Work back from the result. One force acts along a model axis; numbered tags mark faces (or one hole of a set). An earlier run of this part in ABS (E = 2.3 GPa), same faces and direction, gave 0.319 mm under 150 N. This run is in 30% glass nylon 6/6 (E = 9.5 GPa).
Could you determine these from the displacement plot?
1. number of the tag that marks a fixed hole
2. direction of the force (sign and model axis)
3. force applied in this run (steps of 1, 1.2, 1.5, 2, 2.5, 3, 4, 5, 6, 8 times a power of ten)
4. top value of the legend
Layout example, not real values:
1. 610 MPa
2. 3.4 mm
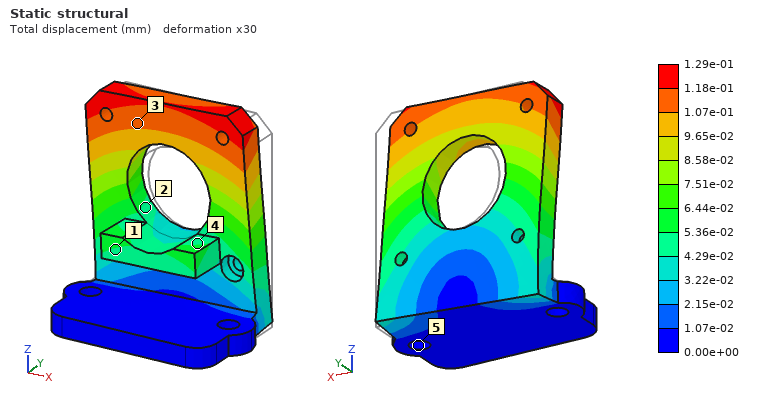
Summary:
1. 5
2. -X
3. 250 N
4. 1.29e-01 mm
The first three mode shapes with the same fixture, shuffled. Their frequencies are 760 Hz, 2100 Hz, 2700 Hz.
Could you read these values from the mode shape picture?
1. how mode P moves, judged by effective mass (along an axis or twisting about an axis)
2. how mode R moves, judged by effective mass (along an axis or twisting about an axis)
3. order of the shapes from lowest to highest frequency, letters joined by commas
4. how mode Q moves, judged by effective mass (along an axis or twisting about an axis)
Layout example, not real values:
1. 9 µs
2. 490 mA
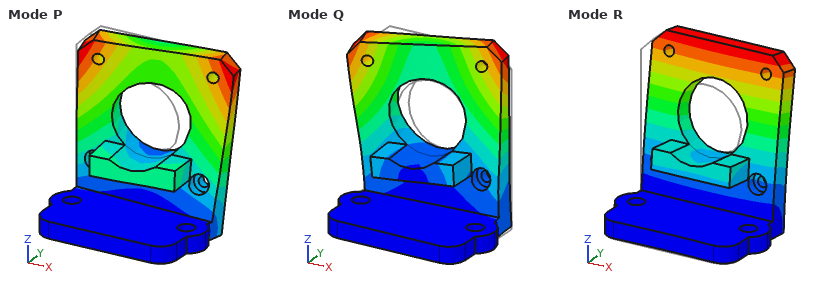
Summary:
1. along X
2. along Y
3. R, P, Q
4. along X
